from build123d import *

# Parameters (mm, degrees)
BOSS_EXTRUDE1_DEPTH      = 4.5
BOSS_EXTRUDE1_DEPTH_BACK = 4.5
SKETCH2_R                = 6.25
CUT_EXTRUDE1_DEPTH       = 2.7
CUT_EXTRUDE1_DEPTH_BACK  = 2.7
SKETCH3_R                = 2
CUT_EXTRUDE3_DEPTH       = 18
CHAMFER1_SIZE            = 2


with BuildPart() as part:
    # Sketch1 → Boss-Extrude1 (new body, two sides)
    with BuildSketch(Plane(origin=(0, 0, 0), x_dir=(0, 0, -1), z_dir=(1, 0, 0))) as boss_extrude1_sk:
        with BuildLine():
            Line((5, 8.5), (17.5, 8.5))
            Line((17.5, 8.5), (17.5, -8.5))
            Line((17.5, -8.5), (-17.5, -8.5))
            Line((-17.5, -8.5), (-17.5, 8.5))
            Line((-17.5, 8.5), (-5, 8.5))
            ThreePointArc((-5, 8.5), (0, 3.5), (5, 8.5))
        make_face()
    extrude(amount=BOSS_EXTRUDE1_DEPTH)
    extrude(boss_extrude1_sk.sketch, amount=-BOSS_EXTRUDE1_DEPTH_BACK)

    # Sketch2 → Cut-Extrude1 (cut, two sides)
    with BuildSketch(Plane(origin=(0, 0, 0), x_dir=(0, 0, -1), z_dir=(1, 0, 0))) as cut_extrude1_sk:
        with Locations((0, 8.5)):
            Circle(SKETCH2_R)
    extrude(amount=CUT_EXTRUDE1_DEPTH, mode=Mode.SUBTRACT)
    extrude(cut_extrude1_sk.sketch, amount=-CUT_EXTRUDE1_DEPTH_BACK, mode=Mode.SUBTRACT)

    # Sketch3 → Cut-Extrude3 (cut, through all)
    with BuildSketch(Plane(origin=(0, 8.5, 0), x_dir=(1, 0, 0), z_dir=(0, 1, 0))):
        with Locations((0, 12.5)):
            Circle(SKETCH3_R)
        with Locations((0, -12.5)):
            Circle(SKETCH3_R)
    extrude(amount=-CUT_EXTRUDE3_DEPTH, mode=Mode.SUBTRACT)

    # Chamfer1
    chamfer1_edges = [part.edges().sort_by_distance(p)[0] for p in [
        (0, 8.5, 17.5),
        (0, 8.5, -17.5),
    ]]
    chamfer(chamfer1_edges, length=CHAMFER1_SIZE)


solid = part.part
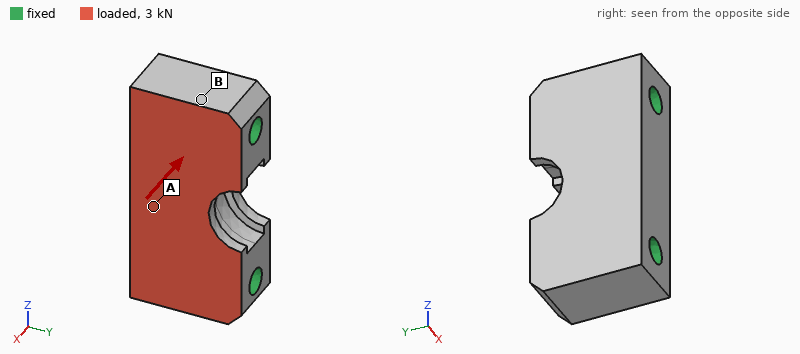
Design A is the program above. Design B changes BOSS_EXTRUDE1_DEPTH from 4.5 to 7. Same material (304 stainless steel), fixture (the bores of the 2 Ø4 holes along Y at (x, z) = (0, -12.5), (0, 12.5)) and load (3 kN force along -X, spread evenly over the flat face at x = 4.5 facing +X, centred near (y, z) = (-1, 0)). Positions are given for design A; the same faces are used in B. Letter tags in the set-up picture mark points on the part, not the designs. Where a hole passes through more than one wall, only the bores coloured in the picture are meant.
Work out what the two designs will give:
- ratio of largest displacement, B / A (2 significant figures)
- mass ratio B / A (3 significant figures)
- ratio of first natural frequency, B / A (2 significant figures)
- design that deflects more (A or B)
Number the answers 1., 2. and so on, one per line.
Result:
1. 0.77
2. 1.31
3. 1.00
4. A
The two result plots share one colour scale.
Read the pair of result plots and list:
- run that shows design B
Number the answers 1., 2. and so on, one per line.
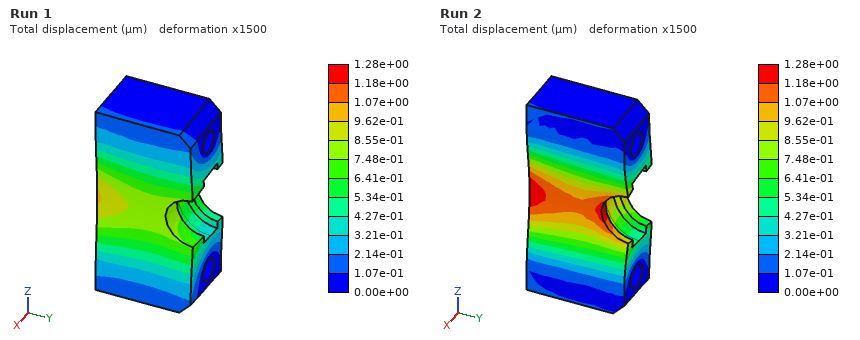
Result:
1. Run 1
